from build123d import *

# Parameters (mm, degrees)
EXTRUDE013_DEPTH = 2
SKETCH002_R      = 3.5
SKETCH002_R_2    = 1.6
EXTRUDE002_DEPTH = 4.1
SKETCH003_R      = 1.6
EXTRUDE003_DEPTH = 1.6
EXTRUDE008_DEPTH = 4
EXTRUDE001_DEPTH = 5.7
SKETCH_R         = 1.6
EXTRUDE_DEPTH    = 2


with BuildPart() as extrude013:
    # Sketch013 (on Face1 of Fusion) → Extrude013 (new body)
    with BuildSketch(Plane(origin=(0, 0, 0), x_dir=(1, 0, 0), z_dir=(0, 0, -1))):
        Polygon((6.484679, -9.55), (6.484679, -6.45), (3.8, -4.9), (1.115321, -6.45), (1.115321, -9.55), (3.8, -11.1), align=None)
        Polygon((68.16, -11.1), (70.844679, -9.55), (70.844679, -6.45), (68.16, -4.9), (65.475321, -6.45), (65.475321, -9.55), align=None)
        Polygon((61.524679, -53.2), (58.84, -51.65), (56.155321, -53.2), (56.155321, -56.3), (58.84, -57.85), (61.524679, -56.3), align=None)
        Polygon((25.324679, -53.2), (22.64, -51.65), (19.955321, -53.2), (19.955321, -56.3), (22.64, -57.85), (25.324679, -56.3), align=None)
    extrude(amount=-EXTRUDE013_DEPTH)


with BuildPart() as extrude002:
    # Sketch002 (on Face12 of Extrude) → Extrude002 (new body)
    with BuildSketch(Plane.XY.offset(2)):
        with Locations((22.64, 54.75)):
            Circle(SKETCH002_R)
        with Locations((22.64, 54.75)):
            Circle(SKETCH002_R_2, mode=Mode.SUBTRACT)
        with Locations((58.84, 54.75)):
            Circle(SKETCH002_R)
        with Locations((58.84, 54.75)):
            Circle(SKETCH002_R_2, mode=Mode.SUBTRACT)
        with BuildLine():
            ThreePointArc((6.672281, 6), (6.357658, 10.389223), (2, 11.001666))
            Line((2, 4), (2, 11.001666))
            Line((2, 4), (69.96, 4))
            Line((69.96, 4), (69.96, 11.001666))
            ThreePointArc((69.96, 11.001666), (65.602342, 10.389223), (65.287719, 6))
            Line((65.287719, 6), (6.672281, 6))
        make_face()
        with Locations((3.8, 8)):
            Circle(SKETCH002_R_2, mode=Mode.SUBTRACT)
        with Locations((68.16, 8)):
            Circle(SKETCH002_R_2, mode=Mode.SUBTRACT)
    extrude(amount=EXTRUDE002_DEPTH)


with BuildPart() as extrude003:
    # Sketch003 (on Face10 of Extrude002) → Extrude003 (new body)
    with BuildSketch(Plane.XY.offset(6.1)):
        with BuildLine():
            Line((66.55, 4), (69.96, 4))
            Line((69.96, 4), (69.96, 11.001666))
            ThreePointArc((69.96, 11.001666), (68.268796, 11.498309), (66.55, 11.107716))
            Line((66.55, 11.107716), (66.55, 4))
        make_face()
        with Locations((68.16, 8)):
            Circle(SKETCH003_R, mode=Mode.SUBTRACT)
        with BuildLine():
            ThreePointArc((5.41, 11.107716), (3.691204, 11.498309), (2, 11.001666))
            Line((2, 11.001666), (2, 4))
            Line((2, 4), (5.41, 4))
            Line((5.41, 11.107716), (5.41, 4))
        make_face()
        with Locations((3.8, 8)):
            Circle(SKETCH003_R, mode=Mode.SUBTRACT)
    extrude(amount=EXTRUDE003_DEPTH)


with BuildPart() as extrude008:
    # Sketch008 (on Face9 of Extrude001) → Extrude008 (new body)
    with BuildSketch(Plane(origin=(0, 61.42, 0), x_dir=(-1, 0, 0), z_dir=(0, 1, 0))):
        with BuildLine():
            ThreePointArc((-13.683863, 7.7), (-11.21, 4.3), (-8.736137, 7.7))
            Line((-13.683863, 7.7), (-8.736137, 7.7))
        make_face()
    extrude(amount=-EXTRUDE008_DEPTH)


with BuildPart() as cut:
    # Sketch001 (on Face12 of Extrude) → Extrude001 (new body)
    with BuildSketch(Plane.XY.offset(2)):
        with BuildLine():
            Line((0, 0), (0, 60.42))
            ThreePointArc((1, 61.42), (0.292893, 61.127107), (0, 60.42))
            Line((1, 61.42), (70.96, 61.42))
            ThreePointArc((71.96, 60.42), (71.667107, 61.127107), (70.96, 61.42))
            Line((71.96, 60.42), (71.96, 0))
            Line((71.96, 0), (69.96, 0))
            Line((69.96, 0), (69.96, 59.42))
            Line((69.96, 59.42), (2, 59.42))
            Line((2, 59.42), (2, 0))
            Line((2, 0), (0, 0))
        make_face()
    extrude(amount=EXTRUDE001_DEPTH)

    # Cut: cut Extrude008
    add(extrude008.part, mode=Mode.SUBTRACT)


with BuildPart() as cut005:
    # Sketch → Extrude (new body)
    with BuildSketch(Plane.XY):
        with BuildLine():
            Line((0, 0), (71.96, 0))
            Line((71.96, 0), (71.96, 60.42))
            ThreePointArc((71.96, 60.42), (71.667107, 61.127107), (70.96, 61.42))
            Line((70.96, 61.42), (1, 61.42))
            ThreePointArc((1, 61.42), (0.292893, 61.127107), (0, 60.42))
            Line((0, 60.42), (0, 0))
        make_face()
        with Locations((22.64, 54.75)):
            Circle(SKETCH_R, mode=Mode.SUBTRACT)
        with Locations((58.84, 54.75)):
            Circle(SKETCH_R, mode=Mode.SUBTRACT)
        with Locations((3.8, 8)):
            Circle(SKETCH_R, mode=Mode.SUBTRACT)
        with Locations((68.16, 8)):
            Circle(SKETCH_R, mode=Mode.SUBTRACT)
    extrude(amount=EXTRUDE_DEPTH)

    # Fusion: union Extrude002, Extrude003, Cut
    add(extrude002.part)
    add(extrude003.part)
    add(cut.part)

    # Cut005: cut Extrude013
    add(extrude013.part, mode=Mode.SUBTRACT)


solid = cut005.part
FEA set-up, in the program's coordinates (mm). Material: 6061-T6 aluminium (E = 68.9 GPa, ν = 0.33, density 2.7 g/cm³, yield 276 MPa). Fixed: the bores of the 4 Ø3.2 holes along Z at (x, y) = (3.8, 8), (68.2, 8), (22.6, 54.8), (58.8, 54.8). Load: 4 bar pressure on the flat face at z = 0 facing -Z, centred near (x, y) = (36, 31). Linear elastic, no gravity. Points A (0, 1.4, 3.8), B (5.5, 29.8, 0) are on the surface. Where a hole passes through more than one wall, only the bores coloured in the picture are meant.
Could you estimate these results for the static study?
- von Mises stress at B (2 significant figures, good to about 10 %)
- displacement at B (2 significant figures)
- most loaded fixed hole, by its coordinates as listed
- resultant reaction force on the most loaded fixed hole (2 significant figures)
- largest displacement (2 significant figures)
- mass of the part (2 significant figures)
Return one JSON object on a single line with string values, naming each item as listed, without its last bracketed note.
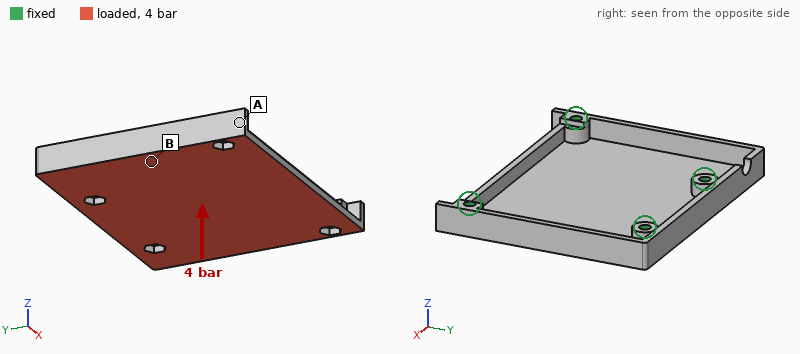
{"von Mises stress at B": "33 MPa", "displacement at B": "0.062 mm", "most loaded fixed hole, by its coordinates as listed": "(3.8, 8)", "resultant reaction force on the most loaded fixed hole": "780 N", "largest displacement": "0.21 mm", "mass of the part": "32 g"}
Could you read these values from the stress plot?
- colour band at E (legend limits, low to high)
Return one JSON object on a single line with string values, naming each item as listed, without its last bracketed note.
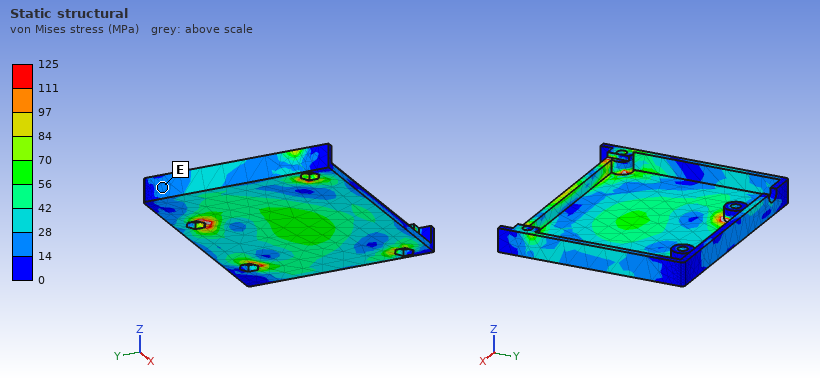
{"colour band at E": "14 to 28 MPa"}
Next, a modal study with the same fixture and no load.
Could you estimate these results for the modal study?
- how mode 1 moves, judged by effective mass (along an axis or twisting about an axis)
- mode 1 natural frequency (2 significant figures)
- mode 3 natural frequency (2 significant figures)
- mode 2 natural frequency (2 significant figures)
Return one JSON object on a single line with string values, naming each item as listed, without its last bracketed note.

{"how mode 1 moves, judged by effective mass": "along Z", "mode 1 natural frequency": "3600 Hz", "mode 3 natural frequency": "6200 Hz", "mode 2 natural frequency": "4800 Hz"}
